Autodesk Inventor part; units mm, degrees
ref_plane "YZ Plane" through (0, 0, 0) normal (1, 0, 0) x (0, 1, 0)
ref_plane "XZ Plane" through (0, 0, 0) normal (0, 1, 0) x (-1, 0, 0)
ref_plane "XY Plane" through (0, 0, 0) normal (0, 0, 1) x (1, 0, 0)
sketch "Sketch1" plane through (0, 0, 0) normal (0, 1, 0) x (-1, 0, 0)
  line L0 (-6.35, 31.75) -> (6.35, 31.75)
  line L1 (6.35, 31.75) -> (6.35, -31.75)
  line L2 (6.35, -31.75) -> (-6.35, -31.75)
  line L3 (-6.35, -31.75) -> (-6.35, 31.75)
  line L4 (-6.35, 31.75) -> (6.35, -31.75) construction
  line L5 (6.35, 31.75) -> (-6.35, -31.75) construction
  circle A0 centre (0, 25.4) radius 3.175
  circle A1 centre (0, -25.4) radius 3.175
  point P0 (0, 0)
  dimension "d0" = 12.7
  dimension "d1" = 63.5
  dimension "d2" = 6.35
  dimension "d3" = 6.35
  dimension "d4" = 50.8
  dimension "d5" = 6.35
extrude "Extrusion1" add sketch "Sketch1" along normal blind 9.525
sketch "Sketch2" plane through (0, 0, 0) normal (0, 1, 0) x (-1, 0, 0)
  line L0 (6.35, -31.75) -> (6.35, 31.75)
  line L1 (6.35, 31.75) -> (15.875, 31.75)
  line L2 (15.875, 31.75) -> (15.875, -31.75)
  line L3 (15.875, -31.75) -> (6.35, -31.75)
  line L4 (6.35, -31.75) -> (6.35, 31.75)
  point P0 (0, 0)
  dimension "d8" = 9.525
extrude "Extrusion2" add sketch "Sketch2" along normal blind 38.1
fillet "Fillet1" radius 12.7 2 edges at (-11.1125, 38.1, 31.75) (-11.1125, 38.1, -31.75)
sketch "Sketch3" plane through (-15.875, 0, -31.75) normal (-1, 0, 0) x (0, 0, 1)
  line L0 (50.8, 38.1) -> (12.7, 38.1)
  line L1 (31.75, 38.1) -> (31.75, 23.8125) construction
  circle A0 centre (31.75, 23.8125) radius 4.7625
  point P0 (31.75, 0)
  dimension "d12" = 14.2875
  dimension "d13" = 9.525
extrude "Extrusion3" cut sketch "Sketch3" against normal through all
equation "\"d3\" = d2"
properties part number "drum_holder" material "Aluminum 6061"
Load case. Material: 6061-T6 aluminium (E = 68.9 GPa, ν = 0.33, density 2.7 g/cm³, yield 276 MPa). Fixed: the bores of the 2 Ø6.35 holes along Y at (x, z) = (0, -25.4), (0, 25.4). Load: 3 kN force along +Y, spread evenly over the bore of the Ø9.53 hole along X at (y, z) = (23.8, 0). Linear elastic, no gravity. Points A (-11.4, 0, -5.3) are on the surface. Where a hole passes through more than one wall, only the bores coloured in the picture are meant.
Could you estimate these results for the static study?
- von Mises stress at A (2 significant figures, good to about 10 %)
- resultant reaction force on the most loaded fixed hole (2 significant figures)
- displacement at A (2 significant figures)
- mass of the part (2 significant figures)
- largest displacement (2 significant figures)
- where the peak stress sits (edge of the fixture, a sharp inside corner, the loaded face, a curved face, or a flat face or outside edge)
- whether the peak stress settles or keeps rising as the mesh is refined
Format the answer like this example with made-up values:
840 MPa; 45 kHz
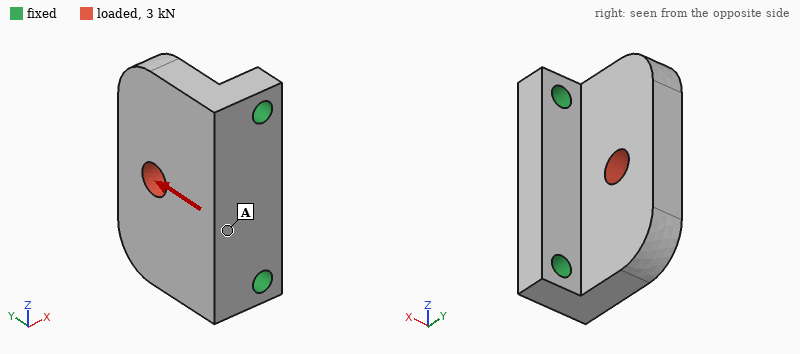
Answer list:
11 MPa; 1.5 kN; 14 µm; 78 g; 40 µm; edge of the fixture; keeps rising
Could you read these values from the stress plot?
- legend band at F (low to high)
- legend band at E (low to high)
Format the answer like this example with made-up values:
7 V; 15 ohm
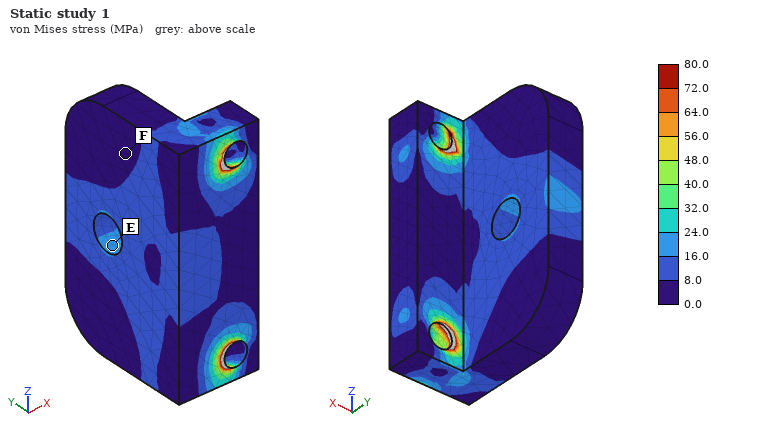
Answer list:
0.0 to 8.0 MPa; 16.0 to 24.0 MPa
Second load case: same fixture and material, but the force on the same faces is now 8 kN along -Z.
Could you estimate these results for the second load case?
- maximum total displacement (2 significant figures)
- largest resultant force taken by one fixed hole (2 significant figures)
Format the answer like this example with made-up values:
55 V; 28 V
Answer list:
42 µm; 5.2 kN
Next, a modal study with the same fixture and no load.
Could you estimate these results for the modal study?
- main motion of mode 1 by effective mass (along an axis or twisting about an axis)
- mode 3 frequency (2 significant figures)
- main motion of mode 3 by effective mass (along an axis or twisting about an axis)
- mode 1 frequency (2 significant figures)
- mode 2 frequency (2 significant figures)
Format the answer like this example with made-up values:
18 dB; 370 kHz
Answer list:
along X; 13 kHz; along Z; 4400 Hz; 8800 Hz
